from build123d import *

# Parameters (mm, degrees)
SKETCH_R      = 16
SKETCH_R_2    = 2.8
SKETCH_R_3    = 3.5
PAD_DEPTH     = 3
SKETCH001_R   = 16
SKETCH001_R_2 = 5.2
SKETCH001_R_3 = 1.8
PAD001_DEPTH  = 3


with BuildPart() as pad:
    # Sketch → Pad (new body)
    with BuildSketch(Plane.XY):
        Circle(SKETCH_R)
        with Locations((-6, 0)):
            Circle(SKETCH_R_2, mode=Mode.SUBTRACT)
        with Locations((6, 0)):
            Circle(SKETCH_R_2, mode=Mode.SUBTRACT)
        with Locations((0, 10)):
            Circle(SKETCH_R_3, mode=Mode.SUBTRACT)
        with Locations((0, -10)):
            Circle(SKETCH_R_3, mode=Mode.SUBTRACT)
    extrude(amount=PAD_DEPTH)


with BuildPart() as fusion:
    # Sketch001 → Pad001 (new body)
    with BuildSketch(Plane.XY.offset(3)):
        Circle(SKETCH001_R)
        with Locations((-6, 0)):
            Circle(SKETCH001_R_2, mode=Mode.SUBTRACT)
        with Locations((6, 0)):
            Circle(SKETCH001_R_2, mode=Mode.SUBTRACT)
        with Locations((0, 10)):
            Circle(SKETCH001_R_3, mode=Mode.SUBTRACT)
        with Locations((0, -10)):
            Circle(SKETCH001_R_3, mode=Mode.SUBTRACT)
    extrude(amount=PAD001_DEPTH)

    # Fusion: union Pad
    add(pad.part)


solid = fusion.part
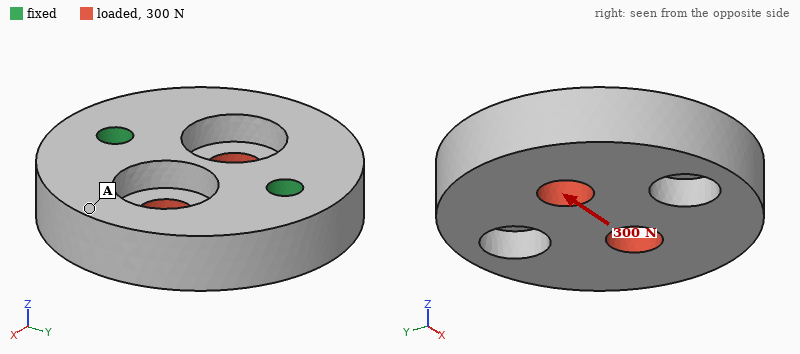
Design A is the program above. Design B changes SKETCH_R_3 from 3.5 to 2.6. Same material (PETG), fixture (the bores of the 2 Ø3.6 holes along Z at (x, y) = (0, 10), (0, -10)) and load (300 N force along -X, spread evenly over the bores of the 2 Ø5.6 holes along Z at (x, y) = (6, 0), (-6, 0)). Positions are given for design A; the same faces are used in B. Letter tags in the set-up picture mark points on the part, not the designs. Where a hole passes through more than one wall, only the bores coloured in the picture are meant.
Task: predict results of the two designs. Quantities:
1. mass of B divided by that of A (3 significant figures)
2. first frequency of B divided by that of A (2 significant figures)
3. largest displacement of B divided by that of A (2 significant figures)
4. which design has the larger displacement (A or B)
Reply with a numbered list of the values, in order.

1. 1.03
2. 1.0
3. 0.87
4. A
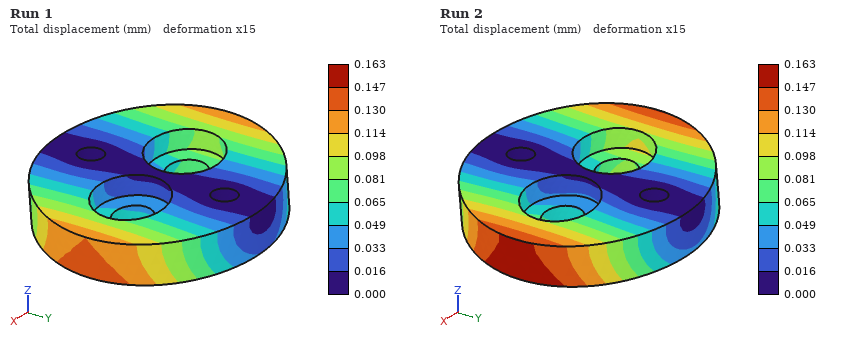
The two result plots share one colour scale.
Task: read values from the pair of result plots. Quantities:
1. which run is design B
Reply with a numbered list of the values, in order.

1. Run 1
